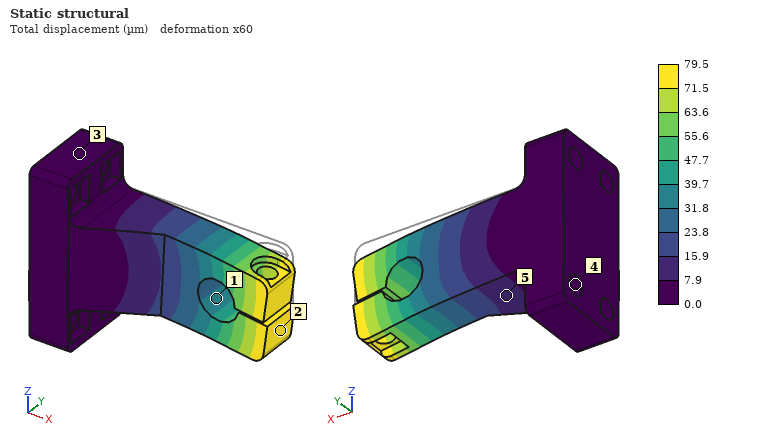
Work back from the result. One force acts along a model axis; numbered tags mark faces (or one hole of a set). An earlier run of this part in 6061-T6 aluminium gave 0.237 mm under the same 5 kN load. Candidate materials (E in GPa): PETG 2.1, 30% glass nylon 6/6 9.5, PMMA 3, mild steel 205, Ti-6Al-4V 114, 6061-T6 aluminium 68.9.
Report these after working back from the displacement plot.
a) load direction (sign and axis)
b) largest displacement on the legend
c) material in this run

-Z
79.5 µm
mild steel
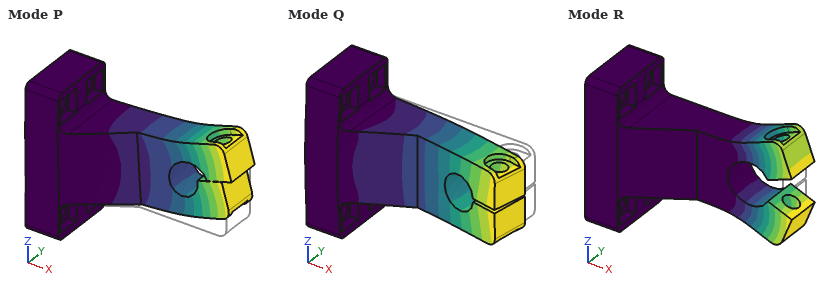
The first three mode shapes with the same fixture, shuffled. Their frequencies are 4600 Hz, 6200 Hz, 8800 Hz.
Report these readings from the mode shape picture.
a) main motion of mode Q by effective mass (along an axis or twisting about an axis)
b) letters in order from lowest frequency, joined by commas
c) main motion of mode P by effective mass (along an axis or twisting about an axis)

along Y
Q, P, R
along Z
